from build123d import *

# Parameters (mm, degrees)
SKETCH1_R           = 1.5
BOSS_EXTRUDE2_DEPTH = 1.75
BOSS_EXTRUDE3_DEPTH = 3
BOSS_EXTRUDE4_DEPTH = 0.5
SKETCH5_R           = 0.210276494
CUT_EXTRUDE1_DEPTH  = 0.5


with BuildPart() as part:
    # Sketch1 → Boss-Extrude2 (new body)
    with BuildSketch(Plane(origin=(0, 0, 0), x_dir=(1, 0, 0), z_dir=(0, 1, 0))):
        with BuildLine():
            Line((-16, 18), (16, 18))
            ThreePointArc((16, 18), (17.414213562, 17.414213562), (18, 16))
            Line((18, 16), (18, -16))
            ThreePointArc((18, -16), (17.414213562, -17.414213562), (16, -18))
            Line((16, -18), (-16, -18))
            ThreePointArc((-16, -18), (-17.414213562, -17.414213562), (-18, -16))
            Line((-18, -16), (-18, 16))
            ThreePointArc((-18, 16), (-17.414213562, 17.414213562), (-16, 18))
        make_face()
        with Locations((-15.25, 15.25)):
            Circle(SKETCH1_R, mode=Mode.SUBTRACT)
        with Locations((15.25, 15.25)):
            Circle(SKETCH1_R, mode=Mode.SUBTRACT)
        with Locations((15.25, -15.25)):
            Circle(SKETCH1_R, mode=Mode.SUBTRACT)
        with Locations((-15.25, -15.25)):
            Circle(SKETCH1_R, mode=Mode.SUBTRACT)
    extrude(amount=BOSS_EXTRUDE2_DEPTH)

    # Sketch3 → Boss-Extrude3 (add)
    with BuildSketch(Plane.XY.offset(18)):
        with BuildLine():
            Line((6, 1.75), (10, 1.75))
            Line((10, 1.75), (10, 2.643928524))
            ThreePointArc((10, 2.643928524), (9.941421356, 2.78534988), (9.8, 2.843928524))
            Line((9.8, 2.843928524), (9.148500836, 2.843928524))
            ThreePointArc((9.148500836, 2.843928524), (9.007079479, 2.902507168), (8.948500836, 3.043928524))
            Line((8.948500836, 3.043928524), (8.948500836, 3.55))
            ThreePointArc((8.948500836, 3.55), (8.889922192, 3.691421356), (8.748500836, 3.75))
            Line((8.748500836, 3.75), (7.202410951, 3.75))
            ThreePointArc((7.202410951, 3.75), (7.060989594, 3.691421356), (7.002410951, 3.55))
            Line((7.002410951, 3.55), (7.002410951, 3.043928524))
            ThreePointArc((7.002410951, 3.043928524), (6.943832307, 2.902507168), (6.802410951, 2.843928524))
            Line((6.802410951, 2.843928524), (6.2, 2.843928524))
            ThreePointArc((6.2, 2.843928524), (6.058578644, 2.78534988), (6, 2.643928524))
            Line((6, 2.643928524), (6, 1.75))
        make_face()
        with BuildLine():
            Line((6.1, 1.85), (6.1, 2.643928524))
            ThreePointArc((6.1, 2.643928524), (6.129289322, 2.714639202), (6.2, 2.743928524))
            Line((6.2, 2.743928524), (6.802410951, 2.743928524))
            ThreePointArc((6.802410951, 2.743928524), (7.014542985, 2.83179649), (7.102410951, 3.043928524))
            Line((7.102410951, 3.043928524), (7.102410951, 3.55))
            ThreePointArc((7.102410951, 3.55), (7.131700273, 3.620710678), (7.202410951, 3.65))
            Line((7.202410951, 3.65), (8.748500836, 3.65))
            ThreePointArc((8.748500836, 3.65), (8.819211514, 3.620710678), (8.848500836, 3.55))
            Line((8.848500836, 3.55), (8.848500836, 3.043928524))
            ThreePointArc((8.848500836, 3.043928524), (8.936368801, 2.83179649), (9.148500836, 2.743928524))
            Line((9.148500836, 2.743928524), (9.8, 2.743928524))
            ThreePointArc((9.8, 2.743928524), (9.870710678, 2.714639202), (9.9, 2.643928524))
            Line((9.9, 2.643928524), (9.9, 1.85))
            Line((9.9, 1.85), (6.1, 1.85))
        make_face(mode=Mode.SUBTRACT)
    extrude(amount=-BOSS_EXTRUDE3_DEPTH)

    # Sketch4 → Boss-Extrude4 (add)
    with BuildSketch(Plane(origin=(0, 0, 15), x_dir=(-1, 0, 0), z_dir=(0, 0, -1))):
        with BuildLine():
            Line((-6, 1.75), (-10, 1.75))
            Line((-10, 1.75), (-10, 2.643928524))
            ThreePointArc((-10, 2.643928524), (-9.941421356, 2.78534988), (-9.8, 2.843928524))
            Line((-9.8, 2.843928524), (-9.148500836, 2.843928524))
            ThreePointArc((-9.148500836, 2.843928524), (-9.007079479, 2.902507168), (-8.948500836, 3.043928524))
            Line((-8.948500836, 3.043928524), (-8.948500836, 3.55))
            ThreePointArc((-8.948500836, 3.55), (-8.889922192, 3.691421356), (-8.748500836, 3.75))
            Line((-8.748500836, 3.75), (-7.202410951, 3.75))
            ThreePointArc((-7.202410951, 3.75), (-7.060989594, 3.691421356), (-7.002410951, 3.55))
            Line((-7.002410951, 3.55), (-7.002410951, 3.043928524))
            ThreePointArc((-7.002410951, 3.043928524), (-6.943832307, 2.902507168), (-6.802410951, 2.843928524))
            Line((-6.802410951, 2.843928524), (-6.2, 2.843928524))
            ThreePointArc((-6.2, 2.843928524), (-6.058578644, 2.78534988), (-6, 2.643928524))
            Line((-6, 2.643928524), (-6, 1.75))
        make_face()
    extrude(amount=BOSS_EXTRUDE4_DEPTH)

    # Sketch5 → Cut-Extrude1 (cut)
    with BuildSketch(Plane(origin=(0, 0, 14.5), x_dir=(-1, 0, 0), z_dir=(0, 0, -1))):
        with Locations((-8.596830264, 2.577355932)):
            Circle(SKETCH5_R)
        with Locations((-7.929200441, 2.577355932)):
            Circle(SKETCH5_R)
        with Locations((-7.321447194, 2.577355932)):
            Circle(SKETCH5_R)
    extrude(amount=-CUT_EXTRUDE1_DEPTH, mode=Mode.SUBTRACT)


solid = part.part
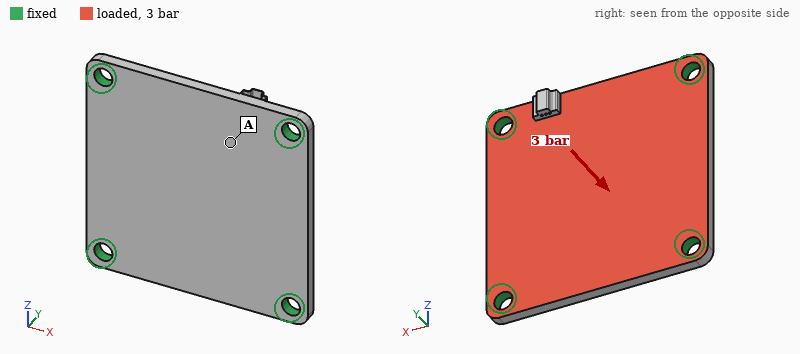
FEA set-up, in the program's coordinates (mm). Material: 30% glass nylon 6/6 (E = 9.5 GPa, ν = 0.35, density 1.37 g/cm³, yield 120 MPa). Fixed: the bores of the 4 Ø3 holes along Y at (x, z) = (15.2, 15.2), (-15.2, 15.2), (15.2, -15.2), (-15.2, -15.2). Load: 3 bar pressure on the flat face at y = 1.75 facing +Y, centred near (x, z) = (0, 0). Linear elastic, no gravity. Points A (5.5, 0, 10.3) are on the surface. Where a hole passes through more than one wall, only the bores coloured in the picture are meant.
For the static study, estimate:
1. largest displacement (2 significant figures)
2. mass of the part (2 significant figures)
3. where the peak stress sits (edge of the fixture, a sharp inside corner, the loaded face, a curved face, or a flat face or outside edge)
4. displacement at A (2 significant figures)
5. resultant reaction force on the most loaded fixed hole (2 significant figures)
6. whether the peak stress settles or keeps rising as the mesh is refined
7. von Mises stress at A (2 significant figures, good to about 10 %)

0.35 mm
3.0 g
edge of the fixture
0.21 mm
95 N
keeps rising
17 MPa
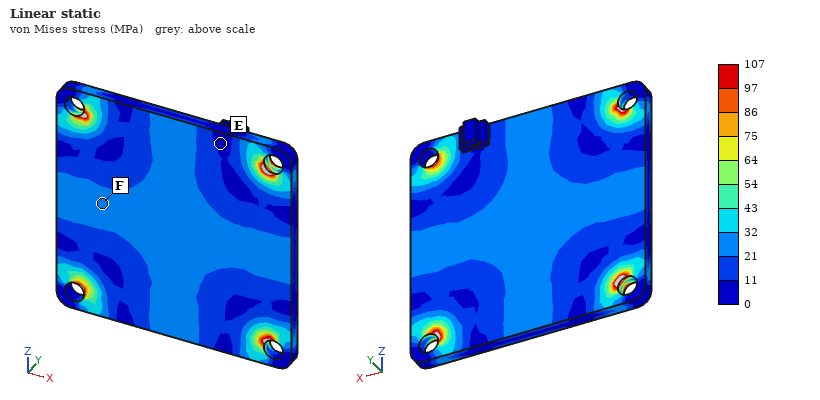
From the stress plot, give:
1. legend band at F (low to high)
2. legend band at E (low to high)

21 to 32 MPa
0 to 11 MPa
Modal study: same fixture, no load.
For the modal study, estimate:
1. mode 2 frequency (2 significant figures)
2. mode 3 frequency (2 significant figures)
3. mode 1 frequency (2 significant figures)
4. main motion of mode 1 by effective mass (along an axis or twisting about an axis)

6100 Hz
6200 Hz
3700 Hz
along Y
